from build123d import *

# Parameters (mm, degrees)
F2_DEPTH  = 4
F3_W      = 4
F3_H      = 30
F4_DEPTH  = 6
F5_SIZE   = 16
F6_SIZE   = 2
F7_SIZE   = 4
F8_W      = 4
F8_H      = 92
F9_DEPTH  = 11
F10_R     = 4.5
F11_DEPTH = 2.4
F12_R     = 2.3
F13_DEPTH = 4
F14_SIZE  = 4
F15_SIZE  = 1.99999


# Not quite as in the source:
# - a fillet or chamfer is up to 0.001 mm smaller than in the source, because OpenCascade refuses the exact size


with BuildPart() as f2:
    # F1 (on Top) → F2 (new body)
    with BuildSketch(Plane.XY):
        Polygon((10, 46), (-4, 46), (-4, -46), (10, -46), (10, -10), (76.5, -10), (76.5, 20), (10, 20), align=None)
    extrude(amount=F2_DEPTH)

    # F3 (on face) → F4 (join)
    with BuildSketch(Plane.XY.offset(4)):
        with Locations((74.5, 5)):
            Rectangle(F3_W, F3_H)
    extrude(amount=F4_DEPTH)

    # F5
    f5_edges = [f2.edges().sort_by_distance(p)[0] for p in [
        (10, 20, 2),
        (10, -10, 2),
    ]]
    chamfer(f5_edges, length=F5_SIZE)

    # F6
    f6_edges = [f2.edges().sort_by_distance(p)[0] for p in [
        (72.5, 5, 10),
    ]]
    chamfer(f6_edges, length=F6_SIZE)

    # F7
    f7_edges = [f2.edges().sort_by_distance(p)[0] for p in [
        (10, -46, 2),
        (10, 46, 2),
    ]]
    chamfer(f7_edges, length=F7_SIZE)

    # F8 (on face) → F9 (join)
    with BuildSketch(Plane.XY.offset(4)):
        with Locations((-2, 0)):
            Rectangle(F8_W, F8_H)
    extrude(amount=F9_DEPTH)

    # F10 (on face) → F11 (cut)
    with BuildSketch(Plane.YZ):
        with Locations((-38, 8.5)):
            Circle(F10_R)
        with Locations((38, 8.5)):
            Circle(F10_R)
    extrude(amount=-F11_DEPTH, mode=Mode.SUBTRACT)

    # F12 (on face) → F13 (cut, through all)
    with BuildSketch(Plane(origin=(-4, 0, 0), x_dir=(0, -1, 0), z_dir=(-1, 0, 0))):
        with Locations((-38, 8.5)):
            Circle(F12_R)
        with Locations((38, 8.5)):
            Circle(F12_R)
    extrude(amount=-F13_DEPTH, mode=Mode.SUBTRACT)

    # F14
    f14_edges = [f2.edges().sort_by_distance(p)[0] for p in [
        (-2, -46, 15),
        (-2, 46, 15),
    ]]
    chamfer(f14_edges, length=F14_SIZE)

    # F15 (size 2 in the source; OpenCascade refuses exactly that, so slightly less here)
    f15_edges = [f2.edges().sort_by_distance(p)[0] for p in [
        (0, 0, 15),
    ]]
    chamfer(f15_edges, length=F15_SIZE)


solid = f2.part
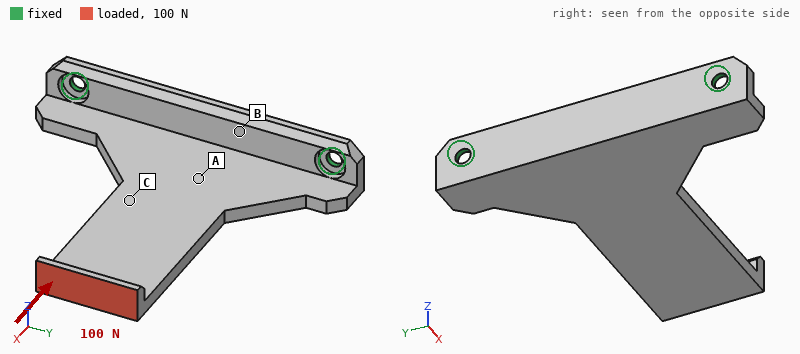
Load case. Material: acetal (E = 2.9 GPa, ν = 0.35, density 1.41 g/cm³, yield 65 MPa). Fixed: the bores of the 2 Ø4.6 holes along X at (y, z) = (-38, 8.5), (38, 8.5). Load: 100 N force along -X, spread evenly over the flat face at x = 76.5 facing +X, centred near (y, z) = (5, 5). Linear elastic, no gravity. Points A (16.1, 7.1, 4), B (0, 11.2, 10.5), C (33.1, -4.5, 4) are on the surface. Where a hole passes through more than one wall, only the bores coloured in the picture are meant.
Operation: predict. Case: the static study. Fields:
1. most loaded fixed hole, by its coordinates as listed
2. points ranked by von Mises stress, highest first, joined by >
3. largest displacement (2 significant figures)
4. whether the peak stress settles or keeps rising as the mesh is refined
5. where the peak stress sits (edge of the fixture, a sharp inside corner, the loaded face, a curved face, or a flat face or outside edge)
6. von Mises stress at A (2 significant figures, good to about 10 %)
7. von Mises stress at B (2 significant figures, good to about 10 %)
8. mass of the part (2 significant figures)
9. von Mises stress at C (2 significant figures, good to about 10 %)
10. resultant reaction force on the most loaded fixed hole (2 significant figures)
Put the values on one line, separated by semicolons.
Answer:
(38, 8.5); C > A > B; 1.4 mm; keeps rising; edge of the fixture; 2.5 MPa; 1.2 MPa; 26 g; 4.6 MPa; 68 N
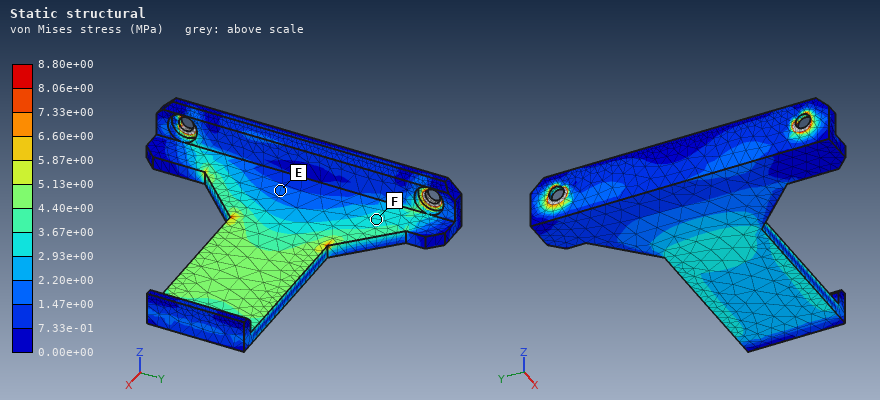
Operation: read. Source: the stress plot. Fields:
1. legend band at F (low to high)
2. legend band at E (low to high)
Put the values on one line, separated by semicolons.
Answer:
2.93e+00 to 3.67e+00 MPa; 1.47e+00 to 2.20e+00 MPa
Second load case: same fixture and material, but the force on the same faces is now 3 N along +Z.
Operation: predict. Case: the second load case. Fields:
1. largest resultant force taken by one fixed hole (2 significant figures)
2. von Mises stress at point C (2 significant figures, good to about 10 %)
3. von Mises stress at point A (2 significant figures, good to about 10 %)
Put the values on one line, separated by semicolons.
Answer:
4.8 N; 1.7 MPa; 1.5 MPa
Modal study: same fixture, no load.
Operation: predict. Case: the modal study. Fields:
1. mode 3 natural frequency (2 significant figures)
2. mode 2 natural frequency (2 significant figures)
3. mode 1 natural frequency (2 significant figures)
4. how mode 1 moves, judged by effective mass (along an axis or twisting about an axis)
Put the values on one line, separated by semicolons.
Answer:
720 Hz; 640 Hz; 110 Hz; along Z
